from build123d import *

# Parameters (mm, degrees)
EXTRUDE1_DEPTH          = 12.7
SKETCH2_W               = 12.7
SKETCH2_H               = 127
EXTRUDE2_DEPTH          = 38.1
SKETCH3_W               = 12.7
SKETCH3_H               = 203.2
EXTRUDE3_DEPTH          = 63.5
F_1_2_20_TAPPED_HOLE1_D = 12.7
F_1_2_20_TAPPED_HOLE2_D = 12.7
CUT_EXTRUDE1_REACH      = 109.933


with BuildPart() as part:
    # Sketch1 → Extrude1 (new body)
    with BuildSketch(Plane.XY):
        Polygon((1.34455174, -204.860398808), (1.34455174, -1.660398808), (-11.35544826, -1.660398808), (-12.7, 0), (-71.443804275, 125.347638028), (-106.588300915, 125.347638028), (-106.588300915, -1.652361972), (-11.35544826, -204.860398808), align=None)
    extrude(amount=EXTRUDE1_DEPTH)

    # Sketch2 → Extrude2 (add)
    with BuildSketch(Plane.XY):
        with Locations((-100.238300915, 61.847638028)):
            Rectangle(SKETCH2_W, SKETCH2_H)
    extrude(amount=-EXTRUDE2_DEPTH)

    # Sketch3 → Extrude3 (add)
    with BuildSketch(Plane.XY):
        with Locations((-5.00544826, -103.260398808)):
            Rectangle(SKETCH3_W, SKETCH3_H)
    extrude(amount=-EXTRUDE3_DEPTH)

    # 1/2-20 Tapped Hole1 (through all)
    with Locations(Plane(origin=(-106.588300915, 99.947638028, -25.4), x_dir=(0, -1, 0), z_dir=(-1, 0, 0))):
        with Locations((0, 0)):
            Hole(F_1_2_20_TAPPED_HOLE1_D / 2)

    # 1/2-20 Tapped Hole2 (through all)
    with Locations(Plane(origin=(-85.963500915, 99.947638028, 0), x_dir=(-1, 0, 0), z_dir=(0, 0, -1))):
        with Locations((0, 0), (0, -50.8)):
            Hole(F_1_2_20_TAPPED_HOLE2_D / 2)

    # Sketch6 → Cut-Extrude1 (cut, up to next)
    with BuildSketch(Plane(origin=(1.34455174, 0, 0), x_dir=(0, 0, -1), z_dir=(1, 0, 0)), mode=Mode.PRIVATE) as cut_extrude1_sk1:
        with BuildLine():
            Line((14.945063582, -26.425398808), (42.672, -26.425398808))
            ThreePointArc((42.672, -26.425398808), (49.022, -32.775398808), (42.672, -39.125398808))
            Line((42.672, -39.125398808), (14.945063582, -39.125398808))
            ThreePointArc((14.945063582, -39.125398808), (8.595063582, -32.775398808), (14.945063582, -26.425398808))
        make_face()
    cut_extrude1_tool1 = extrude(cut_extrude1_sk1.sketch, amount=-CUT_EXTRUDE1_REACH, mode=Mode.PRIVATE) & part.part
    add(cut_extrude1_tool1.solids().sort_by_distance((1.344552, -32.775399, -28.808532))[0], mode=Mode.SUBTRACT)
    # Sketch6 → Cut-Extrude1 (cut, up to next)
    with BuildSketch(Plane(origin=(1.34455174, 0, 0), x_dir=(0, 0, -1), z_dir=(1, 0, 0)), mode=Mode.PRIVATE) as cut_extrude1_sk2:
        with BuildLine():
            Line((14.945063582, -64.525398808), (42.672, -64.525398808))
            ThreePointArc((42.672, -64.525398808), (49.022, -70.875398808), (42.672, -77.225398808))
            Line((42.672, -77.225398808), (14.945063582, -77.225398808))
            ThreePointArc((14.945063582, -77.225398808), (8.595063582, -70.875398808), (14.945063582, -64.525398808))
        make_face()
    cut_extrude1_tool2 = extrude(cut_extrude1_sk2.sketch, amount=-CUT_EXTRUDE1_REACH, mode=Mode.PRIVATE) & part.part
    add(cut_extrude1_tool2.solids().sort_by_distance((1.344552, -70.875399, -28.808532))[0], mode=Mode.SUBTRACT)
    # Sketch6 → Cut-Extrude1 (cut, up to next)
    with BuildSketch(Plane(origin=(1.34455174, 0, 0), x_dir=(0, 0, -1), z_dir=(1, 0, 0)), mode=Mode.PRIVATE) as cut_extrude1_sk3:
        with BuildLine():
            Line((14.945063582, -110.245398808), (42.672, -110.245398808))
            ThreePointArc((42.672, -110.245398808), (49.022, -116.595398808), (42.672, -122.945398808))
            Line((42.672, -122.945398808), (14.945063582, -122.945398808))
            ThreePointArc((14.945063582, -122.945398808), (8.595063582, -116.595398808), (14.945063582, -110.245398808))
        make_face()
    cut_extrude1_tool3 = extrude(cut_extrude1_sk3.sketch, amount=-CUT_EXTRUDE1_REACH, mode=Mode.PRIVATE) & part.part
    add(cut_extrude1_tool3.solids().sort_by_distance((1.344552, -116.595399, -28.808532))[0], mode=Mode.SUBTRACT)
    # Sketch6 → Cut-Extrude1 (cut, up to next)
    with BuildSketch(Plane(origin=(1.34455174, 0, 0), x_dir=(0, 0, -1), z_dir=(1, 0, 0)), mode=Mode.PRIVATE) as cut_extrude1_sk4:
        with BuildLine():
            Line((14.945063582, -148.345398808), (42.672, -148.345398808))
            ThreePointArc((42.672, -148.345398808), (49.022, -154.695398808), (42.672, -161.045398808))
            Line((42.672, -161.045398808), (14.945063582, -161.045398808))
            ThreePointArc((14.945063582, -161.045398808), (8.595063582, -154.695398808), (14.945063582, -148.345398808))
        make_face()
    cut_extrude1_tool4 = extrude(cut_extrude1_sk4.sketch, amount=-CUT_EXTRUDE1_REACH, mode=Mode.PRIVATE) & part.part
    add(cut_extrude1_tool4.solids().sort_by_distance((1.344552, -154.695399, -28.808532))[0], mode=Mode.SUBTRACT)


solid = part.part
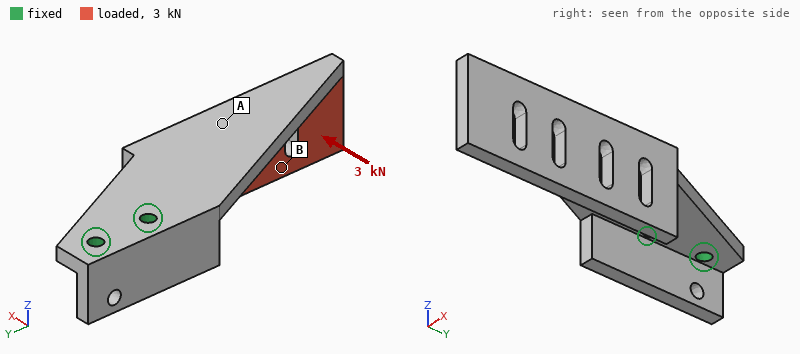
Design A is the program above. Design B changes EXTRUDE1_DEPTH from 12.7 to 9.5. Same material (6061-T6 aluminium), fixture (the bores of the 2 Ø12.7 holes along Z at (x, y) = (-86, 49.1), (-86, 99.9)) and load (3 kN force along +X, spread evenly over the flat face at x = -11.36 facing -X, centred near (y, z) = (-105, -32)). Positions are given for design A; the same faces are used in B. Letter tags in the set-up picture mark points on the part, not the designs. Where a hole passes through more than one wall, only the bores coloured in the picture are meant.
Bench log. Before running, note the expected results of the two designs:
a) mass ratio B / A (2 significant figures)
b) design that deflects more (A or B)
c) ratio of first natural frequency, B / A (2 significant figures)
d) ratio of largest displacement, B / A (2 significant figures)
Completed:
0.86
B
0.72
1.9
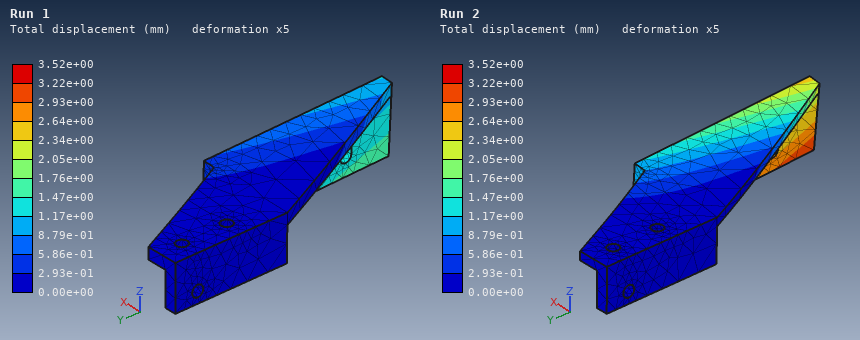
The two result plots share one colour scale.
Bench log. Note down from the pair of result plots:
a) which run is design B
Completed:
Run 2
